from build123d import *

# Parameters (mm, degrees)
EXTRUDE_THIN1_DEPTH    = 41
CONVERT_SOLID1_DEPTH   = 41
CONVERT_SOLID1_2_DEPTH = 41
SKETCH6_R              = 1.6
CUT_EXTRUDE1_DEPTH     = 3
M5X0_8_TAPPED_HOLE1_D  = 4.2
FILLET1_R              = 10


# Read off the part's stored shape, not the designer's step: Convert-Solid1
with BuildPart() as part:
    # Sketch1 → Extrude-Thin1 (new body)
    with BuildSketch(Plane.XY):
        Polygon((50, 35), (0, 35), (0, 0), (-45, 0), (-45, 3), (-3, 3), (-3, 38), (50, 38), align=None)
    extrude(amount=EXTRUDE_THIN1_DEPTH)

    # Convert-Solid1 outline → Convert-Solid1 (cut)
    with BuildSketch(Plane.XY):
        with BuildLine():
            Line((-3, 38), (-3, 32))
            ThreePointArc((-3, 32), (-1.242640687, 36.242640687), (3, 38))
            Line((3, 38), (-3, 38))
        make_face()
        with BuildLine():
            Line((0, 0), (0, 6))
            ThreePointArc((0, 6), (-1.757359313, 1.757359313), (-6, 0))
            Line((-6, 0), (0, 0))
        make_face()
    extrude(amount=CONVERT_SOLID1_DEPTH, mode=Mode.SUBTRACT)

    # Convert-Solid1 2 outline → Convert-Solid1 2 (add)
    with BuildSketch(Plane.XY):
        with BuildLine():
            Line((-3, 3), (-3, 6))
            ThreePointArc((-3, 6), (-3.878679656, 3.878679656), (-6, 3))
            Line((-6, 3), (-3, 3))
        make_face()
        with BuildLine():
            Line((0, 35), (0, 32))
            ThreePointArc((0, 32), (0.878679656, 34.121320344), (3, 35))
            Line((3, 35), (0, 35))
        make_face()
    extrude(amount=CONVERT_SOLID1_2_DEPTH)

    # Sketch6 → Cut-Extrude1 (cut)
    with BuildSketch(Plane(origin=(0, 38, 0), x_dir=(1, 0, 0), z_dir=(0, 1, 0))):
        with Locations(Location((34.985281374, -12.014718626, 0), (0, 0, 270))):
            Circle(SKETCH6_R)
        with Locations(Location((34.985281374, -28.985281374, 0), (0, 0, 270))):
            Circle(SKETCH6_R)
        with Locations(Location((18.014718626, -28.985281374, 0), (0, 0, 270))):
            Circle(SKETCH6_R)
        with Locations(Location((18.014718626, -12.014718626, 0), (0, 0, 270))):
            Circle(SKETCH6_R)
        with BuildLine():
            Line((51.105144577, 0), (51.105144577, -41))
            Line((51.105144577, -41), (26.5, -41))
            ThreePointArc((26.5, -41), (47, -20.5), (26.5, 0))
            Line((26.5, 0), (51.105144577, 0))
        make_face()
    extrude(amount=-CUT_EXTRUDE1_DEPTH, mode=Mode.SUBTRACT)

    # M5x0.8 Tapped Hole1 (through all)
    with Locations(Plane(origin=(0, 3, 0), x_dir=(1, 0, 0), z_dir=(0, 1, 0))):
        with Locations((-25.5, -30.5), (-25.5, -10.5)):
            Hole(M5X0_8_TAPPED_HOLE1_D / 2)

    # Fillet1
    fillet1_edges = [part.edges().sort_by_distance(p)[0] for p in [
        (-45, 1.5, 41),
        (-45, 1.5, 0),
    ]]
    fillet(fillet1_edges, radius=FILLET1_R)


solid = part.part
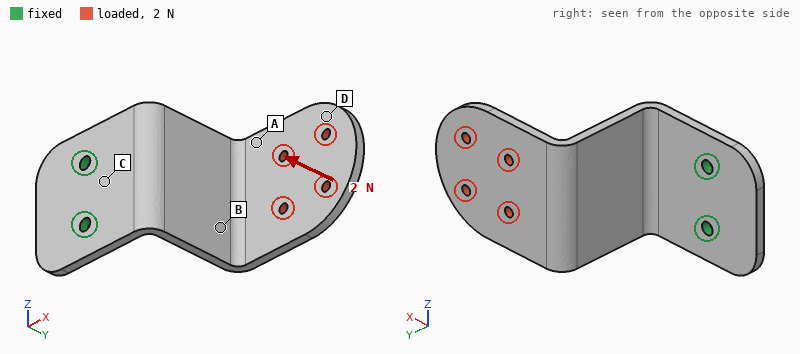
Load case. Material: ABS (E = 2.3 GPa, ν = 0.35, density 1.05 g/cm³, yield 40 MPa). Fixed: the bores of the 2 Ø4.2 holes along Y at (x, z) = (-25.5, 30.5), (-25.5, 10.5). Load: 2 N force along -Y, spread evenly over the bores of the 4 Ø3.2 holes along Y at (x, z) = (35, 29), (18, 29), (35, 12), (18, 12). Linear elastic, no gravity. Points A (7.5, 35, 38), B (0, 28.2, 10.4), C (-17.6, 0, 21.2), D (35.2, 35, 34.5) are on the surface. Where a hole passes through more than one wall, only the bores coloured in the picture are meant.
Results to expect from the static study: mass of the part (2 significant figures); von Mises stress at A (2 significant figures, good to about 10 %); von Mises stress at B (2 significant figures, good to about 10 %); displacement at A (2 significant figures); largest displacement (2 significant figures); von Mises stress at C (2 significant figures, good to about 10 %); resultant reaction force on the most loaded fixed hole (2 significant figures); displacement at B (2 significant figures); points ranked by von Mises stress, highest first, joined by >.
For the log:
15 g
0.55 MPa
0.84 MPa
0.47 mm
1.1 mm
1.2 MPa
1.0 N
0.32 mm
C > B > A > D
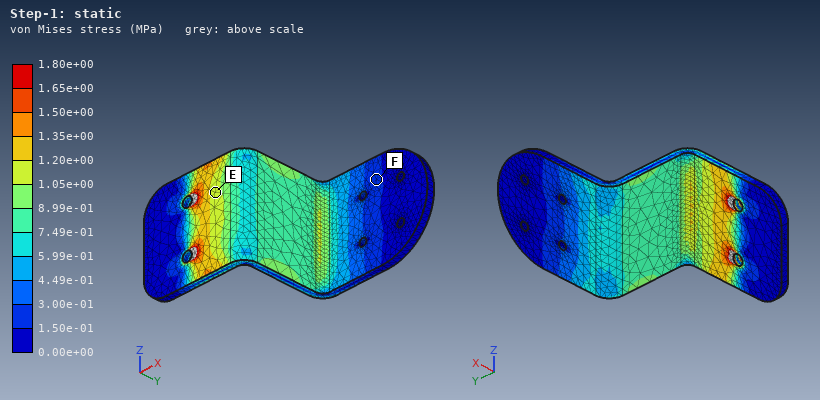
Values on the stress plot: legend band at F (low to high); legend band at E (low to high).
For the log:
1.50e-01 to 3.00e-01 MPa
1.05e+00 to 1.20e+00 MPa
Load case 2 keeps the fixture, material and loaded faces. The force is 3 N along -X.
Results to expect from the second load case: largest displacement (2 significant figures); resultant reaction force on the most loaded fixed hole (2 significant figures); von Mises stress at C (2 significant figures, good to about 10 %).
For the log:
1.1 mm
1.6 N
1.5 MPa
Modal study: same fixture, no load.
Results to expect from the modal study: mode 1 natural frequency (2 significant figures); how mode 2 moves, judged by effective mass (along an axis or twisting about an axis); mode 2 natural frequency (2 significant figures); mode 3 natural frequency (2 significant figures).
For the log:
100 Hz
along Z
240 Hz
370 Hz
